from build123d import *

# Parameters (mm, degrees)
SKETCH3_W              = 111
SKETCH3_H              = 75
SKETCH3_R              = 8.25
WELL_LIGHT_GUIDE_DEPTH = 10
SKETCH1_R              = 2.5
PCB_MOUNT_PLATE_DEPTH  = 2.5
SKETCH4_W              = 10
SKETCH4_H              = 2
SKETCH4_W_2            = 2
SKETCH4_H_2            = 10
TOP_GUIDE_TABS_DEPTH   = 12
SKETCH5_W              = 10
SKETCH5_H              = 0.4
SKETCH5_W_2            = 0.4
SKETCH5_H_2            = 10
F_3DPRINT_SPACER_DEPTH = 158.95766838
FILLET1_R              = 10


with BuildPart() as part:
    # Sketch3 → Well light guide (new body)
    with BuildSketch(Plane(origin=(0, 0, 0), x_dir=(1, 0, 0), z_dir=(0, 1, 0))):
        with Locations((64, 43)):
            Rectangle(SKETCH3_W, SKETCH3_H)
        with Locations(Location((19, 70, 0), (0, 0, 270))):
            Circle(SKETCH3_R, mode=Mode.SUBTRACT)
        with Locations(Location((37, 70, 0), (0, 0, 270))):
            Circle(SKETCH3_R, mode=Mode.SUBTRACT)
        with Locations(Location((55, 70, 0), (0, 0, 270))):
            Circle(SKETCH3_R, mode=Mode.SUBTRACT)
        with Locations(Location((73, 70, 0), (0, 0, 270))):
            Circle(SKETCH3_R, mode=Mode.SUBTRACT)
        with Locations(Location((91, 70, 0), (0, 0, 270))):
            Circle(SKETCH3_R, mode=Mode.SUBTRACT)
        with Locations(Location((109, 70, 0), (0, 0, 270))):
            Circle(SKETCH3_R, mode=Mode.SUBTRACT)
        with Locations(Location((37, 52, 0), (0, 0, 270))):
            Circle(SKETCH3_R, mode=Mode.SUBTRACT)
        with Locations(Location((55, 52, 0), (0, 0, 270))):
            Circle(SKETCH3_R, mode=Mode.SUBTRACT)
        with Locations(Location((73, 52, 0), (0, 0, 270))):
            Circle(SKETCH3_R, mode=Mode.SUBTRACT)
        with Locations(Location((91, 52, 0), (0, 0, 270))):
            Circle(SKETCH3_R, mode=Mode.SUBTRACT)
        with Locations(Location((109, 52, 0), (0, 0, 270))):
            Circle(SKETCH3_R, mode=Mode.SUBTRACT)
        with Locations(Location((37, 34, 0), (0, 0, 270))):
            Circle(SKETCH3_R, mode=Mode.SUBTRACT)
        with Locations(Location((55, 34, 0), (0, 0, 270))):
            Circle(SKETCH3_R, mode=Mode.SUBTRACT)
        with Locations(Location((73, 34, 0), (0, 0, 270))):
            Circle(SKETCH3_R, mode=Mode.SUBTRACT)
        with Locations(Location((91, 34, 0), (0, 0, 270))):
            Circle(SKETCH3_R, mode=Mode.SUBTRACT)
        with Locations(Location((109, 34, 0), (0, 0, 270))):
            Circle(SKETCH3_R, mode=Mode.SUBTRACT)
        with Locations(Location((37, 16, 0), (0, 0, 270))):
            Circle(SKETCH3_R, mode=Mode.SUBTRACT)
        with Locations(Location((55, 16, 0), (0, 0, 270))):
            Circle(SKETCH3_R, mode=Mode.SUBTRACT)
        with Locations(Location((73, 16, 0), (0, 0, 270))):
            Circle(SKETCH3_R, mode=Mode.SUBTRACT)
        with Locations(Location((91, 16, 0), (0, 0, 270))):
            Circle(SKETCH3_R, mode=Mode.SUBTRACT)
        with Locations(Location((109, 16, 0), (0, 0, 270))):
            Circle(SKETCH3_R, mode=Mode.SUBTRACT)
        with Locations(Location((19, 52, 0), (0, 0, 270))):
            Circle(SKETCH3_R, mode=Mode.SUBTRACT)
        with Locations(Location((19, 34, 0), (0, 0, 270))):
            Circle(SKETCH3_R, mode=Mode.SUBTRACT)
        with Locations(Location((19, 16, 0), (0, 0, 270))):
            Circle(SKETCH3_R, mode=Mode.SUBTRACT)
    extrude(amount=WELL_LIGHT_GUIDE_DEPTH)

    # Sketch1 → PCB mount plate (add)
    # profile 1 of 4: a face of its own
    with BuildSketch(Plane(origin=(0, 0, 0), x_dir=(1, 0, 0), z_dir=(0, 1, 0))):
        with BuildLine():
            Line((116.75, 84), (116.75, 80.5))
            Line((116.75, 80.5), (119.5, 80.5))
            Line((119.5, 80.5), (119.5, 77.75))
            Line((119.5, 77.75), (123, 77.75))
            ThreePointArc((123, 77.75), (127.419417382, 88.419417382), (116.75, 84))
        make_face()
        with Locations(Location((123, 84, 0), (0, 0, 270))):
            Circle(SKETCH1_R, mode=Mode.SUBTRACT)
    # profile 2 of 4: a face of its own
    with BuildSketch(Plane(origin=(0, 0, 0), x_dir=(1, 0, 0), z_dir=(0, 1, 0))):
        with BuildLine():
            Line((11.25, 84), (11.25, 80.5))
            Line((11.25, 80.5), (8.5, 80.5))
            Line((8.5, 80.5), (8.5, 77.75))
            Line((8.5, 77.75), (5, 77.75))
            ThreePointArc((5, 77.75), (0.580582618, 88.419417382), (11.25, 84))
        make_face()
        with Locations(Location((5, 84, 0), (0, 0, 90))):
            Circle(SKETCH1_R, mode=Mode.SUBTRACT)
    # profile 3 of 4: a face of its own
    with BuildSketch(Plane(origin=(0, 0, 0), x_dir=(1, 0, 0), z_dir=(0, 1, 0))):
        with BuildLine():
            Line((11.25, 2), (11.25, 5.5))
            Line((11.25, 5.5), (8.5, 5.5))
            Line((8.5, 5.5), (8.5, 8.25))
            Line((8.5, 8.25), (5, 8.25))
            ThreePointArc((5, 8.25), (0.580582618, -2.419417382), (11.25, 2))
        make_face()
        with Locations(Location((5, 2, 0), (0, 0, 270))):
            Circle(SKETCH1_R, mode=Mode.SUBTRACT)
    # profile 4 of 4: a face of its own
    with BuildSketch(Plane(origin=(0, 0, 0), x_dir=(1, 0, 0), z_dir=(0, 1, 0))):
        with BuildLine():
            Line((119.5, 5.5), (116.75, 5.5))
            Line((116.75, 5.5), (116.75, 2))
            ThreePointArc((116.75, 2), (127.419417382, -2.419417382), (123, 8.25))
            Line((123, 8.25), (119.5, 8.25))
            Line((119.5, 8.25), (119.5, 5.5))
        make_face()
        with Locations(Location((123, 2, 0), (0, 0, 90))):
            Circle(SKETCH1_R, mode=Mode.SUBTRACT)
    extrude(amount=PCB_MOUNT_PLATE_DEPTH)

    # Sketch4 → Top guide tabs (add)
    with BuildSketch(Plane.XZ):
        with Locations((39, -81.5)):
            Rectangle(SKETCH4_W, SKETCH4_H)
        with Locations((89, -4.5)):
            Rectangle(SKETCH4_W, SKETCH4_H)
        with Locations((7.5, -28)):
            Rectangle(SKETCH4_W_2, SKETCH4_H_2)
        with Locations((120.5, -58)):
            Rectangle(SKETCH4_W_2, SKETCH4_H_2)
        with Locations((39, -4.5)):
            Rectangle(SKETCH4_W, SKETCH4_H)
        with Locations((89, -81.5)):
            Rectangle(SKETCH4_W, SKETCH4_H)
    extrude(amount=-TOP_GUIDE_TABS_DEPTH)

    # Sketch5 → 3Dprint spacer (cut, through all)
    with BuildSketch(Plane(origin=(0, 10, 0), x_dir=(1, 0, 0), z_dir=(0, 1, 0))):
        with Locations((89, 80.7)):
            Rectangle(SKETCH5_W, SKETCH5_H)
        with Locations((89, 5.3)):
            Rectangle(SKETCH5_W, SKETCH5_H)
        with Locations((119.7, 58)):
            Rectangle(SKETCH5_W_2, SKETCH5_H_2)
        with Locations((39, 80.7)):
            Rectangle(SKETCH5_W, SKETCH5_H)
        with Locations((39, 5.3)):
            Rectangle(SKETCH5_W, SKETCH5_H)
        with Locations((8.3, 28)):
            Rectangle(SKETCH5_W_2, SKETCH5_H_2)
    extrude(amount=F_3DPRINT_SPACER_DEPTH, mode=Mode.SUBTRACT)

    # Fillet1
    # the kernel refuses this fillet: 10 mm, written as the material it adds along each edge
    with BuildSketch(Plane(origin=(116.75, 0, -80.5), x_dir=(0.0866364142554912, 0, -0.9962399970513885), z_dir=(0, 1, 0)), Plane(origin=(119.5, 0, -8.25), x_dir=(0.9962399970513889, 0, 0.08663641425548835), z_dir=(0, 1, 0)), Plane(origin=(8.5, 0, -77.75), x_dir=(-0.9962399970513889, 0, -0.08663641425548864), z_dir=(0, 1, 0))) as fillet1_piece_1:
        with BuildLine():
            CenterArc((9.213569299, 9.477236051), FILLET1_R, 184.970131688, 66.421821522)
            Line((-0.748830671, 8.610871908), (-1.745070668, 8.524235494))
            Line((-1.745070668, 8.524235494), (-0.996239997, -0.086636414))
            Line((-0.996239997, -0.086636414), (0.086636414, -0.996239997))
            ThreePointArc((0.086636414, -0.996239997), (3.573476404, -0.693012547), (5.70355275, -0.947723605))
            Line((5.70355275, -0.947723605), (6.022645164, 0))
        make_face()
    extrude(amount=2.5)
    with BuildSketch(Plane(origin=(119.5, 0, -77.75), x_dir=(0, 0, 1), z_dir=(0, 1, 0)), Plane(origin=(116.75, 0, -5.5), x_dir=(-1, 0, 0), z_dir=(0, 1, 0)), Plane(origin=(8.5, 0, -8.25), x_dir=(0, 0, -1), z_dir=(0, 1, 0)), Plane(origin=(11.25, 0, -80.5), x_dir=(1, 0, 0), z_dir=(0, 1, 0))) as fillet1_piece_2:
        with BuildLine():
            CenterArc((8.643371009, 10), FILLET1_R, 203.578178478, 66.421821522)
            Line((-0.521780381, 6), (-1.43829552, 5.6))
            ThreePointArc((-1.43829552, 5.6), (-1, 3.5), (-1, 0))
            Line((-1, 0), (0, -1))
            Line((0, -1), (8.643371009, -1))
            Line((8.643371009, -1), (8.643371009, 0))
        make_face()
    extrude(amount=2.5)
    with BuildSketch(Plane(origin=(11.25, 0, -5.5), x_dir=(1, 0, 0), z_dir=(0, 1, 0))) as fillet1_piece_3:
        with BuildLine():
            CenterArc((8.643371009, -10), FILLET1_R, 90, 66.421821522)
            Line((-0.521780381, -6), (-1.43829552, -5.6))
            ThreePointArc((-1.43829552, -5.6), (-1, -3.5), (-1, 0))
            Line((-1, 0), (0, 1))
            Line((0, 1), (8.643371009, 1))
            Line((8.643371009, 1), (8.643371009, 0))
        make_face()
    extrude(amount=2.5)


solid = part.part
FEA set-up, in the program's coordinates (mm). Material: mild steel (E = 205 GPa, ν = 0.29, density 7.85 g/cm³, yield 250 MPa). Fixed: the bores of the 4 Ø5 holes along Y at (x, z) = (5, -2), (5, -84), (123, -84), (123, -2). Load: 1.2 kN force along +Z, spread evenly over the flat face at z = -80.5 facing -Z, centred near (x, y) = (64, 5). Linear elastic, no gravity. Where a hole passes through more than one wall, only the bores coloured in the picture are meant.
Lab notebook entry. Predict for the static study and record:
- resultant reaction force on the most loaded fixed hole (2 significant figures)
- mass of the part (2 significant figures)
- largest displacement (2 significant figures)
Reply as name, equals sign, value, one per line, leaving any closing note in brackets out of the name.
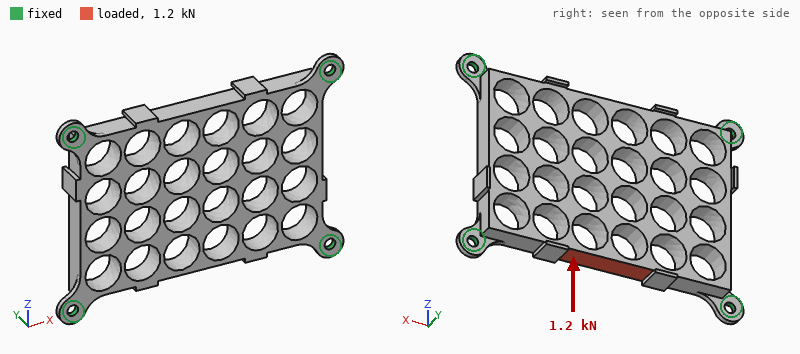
resultant reaction force on the most loaded fixed hole = 350 N
mass of the part = 270 g
largest displacement = 23 µm
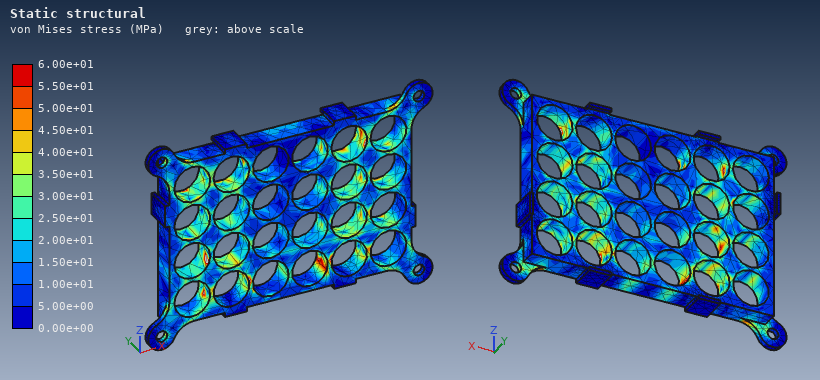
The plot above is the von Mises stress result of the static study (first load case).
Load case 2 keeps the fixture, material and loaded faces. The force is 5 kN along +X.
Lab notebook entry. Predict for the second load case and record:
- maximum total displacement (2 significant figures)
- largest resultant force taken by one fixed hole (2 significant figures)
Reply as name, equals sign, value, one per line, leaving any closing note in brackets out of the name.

maximum total displacement = 32 µm
largest resultant force taken by one fixed hole = 2.2 kN
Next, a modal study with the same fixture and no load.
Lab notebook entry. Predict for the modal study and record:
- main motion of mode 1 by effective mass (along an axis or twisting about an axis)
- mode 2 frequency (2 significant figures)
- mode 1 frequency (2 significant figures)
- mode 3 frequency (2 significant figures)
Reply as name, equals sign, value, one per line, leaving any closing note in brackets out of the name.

main motion of mode 1 by effective mass = along Y
mode 2 frequency = 2300 Hz
mode 1 frequency = 1600 Hz
mode 3 frequency = 3400 Hz
